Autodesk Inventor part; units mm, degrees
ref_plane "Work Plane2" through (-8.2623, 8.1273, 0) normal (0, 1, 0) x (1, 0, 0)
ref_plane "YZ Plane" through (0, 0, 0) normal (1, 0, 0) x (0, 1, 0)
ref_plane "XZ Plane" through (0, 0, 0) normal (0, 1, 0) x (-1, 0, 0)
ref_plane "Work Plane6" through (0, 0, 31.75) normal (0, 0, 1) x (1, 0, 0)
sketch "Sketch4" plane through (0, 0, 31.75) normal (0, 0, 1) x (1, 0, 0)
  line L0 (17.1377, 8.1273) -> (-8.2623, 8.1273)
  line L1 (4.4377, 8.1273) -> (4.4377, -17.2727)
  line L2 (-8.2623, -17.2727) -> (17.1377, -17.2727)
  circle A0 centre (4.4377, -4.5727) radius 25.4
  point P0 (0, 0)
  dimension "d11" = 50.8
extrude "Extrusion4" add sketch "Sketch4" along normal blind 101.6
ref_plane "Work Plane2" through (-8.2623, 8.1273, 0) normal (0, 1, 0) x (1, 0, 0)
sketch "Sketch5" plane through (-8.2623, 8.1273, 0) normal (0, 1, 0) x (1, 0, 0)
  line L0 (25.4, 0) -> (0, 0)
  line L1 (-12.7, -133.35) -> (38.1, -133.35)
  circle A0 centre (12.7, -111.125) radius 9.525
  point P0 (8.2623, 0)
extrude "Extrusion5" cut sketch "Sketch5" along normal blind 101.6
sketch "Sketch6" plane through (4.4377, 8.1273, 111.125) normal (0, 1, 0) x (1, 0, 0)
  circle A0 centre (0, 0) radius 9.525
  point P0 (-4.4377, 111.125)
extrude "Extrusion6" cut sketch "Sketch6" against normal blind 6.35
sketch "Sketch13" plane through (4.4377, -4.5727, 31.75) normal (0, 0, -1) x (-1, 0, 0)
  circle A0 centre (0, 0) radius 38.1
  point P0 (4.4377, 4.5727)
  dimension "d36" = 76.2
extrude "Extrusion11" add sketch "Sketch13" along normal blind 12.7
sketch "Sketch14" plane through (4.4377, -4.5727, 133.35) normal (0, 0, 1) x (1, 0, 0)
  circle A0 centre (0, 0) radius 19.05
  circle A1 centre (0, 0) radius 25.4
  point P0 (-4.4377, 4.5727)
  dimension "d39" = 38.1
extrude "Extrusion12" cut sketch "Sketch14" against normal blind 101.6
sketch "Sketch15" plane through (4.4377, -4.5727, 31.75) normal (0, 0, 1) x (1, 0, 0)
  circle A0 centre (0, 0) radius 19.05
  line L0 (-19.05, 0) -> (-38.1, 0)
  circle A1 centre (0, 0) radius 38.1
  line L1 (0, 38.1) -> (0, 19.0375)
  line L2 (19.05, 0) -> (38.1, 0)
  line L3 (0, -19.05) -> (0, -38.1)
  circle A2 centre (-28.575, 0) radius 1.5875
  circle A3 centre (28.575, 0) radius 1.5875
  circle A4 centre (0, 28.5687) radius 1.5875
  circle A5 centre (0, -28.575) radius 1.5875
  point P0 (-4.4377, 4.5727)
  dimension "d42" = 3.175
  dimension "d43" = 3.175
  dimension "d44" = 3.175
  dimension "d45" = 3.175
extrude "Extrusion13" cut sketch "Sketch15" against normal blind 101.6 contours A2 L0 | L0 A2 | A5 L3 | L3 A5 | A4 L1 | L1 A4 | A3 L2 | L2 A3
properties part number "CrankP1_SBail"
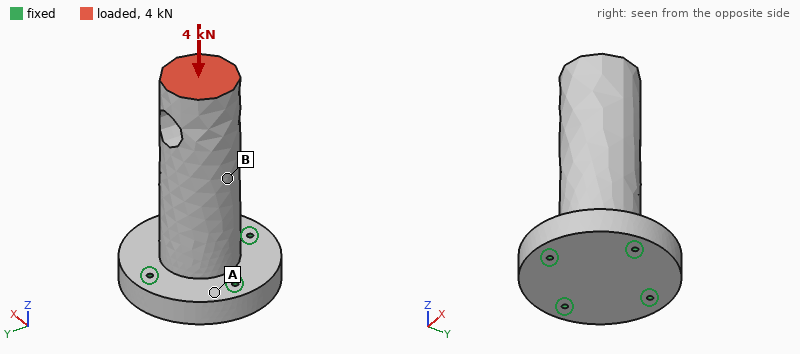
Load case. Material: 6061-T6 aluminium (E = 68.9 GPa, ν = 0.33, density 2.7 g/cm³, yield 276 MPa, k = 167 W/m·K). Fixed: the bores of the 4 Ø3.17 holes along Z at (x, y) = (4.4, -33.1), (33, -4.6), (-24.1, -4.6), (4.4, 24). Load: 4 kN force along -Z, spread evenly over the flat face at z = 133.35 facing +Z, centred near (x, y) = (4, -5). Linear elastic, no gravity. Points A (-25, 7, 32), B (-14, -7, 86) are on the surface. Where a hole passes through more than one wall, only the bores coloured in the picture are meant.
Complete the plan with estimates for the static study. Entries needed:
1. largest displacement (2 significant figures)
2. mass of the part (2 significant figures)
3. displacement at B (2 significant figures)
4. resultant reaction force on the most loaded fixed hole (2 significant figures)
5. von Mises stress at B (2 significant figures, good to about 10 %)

12 µm
460 g
6.3 µm
1.0 kN
4.0 MPa
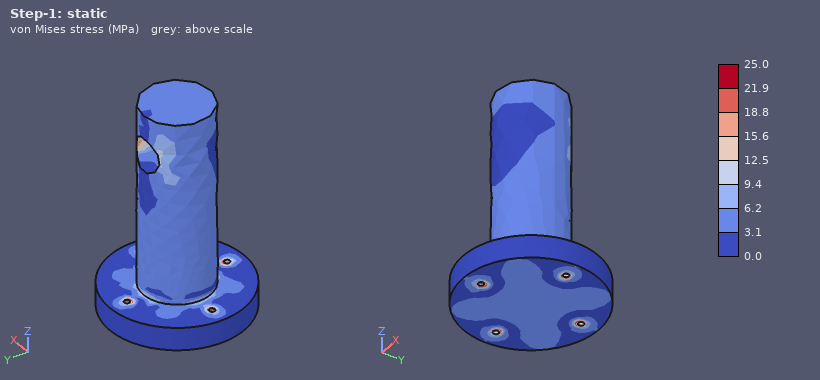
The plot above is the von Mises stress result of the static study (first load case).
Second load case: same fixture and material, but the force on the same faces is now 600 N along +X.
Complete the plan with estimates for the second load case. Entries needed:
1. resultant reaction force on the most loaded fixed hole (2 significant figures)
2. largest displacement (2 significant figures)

1.1 kN
52 µm
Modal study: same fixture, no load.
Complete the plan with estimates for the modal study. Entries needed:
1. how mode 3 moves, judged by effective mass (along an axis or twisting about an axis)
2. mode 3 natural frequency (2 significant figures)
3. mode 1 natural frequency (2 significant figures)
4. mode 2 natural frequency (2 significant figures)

twisting about Z
7300 Hz
1900 Hz
1900 Hz
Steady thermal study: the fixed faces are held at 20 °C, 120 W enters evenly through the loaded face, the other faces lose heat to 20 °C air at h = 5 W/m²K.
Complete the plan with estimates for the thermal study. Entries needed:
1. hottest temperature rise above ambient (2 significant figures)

79 K
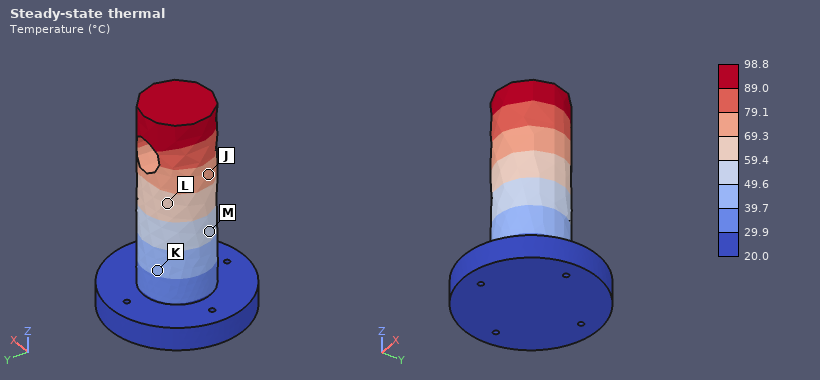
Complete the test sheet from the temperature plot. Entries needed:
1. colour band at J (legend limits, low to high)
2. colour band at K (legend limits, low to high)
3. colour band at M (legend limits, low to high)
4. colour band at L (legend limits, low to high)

69.3 to 79.1 °C
39.7 to 49.6 °C
49.6 to 59.4 °C
59.4 to 69.3 °C
